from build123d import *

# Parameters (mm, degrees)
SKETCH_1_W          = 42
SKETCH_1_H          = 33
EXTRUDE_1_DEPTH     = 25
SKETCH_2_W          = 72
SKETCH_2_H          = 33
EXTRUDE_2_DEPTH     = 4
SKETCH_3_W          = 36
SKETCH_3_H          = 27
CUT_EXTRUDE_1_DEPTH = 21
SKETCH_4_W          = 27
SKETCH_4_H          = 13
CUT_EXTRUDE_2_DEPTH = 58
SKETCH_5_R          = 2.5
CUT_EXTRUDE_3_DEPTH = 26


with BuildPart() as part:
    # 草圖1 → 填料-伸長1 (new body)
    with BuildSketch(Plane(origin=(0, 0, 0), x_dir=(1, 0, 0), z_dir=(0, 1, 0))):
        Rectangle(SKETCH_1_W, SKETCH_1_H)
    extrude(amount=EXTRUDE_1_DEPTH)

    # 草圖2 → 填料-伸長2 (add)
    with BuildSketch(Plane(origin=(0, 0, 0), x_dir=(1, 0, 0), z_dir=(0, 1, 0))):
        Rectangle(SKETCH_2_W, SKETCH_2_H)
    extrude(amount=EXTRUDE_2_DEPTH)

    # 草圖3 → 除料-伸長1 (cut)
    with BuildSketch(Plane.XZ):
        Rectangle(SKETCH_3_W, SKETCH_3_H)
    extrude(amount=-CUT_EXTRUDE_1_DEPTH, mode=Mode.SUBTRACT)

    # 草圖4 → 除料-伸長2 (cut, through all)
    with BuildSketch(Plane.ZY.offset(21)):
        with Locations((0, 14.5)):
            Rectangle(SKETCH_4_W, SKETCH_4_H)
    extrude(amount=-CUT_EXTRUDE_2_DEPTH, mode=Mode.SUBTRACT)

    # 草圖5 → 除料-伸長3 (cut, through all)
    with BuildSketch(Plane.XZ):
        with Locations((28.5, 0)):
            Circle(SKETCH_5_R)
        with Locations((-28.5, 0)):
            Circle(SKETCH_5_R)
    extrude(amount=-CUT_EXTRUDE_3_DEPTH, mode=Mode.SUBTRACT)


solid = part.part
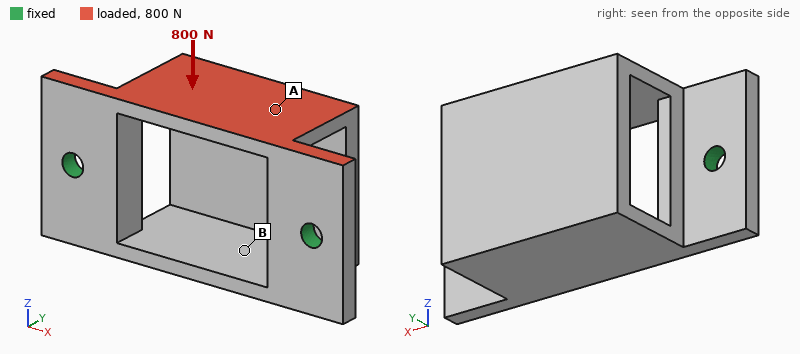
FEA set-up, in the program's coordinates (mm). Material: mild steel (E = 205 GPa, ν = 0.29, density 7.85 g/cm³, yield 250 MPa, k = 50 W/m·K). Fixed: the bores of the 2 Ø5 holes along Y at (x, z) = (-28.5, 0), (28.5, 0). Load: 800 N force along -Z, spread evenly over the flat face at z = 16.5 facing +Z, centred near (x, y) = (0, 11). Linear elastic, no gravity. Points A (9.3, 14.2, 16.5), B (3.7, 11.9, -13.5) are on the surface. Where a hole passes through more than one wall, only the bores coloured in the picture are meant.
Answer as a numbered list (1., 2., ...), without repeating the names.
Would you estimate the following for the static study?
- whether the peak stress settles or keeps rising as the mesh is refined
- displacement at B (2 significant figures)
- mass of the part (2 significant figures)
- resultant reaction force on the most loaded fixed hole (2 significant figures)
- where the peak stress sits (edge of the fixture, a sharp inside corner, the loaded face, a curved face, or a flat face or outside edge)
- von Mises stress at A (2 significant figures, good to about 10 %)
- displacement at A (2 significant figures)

1. keeps rising
2. 16 µm
3. 130 g
4. 410 N
5. edge of the fixture
6. 22 MPa
7. 23 µm
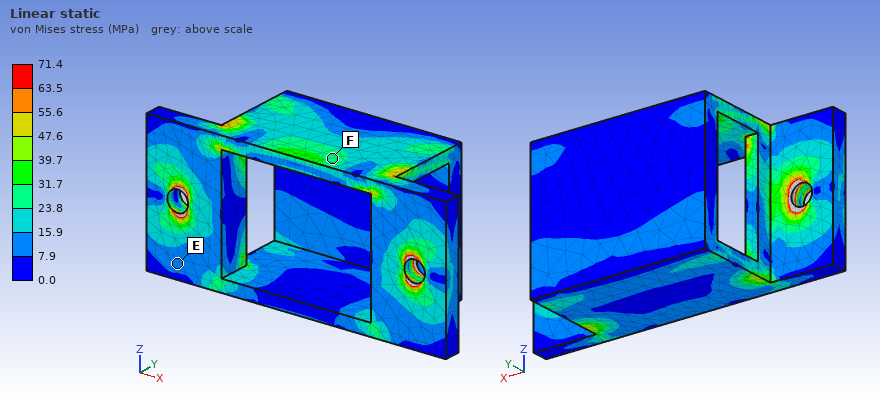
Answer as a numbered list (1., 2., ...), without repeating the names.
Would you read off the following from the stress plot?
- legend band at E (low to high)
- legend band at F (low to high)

1. 7.9 to 15.9 MPa
2. 23.8 to 31.7 MPa
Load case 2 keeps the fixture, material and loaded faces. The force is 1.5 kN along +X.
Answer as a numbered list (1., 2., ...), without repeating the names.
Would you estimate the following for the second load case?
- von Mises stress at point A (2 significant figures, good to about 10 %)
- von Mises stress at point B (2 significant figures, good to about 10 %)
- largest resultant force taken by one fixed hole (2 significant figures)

1. 23 MPa
2. 12 MPa
3. 830 N
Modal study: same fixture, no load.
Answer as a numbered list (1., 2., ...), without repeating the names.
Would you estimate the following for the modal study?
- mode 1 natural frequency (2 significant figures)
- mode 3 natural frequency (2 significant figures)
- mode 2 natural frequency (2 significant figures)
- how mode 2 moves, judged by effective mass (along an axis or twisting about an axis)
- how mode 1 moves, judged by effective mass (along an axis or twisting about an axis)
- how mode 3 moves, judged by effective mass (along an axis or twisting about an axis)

1. 2300 Hz
2. 6300 Hz
3. 5500 Hz
4. along Y
5. along Z
6. along X
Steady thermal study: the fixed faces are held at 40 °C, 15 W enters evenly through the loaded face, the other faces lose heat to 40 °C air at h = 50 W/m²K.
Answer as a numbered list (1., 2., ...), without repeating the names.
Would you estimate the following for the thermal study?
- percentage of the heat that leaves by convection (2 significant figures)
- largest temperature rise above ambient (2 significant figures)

1. 44 %
2. 35 K
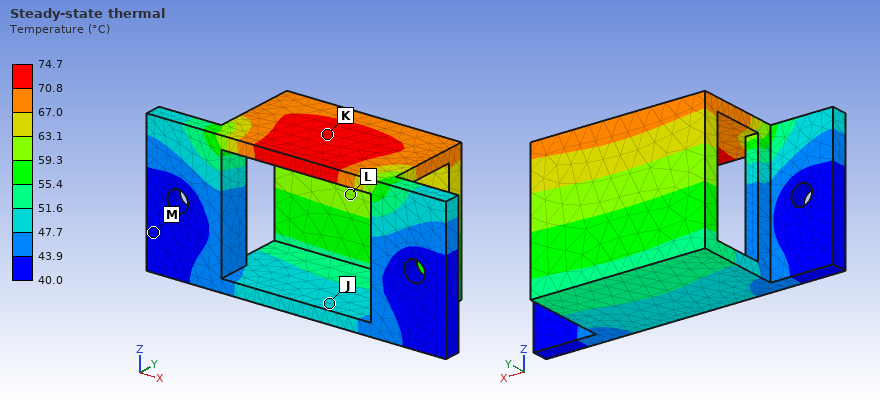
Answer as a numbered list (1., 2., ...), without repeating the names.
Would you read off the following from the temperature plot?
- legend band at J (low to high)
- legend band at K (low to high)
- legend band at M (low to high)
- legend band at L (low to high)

1. 47.7 to 51.6 °C
2. 70.8 to 74.7 °C
3. 40.0 to 43.9 °C
4. 59.3 to 63.1 °C
